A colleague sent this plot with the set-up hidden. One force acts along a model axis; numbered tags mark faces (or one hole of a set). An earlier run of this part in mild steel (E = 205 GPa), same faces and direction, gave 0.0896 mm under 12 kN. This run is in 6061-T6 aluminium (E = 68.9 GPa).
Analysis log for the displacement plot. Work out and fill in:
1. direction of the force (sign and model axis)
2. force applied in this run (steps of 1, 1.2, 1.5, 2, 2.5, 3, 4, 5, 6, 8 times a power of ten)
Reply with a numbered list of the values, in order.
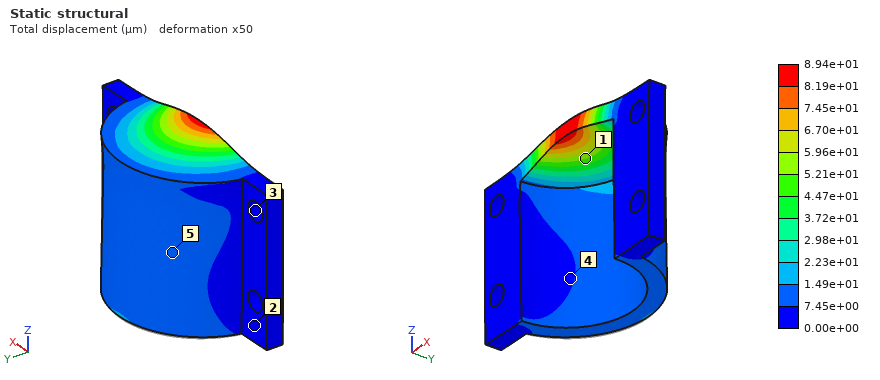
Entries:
1. +Z
2. 4 kN
